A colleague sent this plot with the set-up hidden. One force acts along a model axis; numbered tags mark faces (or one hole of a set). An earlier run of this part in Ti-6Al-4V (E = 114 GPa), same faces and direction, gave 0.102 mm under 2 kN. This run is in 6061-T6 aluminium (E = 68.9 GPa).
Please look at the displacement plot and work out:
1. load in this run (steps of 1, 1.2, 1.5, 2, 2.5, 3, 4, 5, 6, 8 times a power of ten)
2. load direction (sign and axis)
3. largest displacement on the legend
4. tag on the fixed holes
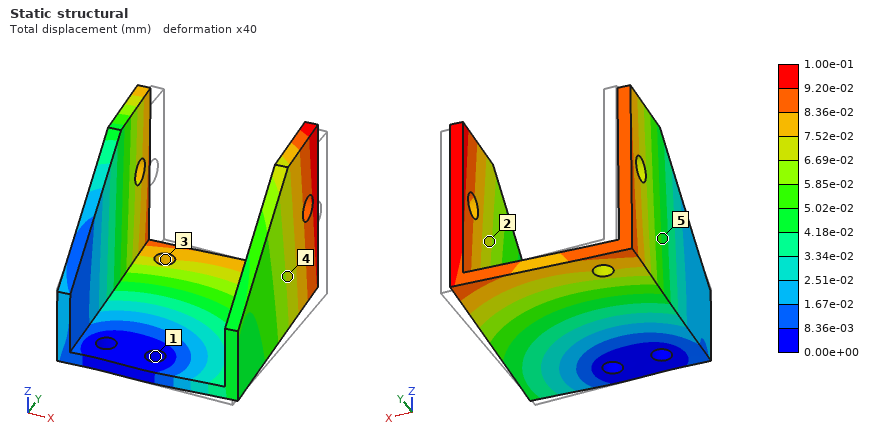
1.2 kN
-X
1.00e-01 mm
1
